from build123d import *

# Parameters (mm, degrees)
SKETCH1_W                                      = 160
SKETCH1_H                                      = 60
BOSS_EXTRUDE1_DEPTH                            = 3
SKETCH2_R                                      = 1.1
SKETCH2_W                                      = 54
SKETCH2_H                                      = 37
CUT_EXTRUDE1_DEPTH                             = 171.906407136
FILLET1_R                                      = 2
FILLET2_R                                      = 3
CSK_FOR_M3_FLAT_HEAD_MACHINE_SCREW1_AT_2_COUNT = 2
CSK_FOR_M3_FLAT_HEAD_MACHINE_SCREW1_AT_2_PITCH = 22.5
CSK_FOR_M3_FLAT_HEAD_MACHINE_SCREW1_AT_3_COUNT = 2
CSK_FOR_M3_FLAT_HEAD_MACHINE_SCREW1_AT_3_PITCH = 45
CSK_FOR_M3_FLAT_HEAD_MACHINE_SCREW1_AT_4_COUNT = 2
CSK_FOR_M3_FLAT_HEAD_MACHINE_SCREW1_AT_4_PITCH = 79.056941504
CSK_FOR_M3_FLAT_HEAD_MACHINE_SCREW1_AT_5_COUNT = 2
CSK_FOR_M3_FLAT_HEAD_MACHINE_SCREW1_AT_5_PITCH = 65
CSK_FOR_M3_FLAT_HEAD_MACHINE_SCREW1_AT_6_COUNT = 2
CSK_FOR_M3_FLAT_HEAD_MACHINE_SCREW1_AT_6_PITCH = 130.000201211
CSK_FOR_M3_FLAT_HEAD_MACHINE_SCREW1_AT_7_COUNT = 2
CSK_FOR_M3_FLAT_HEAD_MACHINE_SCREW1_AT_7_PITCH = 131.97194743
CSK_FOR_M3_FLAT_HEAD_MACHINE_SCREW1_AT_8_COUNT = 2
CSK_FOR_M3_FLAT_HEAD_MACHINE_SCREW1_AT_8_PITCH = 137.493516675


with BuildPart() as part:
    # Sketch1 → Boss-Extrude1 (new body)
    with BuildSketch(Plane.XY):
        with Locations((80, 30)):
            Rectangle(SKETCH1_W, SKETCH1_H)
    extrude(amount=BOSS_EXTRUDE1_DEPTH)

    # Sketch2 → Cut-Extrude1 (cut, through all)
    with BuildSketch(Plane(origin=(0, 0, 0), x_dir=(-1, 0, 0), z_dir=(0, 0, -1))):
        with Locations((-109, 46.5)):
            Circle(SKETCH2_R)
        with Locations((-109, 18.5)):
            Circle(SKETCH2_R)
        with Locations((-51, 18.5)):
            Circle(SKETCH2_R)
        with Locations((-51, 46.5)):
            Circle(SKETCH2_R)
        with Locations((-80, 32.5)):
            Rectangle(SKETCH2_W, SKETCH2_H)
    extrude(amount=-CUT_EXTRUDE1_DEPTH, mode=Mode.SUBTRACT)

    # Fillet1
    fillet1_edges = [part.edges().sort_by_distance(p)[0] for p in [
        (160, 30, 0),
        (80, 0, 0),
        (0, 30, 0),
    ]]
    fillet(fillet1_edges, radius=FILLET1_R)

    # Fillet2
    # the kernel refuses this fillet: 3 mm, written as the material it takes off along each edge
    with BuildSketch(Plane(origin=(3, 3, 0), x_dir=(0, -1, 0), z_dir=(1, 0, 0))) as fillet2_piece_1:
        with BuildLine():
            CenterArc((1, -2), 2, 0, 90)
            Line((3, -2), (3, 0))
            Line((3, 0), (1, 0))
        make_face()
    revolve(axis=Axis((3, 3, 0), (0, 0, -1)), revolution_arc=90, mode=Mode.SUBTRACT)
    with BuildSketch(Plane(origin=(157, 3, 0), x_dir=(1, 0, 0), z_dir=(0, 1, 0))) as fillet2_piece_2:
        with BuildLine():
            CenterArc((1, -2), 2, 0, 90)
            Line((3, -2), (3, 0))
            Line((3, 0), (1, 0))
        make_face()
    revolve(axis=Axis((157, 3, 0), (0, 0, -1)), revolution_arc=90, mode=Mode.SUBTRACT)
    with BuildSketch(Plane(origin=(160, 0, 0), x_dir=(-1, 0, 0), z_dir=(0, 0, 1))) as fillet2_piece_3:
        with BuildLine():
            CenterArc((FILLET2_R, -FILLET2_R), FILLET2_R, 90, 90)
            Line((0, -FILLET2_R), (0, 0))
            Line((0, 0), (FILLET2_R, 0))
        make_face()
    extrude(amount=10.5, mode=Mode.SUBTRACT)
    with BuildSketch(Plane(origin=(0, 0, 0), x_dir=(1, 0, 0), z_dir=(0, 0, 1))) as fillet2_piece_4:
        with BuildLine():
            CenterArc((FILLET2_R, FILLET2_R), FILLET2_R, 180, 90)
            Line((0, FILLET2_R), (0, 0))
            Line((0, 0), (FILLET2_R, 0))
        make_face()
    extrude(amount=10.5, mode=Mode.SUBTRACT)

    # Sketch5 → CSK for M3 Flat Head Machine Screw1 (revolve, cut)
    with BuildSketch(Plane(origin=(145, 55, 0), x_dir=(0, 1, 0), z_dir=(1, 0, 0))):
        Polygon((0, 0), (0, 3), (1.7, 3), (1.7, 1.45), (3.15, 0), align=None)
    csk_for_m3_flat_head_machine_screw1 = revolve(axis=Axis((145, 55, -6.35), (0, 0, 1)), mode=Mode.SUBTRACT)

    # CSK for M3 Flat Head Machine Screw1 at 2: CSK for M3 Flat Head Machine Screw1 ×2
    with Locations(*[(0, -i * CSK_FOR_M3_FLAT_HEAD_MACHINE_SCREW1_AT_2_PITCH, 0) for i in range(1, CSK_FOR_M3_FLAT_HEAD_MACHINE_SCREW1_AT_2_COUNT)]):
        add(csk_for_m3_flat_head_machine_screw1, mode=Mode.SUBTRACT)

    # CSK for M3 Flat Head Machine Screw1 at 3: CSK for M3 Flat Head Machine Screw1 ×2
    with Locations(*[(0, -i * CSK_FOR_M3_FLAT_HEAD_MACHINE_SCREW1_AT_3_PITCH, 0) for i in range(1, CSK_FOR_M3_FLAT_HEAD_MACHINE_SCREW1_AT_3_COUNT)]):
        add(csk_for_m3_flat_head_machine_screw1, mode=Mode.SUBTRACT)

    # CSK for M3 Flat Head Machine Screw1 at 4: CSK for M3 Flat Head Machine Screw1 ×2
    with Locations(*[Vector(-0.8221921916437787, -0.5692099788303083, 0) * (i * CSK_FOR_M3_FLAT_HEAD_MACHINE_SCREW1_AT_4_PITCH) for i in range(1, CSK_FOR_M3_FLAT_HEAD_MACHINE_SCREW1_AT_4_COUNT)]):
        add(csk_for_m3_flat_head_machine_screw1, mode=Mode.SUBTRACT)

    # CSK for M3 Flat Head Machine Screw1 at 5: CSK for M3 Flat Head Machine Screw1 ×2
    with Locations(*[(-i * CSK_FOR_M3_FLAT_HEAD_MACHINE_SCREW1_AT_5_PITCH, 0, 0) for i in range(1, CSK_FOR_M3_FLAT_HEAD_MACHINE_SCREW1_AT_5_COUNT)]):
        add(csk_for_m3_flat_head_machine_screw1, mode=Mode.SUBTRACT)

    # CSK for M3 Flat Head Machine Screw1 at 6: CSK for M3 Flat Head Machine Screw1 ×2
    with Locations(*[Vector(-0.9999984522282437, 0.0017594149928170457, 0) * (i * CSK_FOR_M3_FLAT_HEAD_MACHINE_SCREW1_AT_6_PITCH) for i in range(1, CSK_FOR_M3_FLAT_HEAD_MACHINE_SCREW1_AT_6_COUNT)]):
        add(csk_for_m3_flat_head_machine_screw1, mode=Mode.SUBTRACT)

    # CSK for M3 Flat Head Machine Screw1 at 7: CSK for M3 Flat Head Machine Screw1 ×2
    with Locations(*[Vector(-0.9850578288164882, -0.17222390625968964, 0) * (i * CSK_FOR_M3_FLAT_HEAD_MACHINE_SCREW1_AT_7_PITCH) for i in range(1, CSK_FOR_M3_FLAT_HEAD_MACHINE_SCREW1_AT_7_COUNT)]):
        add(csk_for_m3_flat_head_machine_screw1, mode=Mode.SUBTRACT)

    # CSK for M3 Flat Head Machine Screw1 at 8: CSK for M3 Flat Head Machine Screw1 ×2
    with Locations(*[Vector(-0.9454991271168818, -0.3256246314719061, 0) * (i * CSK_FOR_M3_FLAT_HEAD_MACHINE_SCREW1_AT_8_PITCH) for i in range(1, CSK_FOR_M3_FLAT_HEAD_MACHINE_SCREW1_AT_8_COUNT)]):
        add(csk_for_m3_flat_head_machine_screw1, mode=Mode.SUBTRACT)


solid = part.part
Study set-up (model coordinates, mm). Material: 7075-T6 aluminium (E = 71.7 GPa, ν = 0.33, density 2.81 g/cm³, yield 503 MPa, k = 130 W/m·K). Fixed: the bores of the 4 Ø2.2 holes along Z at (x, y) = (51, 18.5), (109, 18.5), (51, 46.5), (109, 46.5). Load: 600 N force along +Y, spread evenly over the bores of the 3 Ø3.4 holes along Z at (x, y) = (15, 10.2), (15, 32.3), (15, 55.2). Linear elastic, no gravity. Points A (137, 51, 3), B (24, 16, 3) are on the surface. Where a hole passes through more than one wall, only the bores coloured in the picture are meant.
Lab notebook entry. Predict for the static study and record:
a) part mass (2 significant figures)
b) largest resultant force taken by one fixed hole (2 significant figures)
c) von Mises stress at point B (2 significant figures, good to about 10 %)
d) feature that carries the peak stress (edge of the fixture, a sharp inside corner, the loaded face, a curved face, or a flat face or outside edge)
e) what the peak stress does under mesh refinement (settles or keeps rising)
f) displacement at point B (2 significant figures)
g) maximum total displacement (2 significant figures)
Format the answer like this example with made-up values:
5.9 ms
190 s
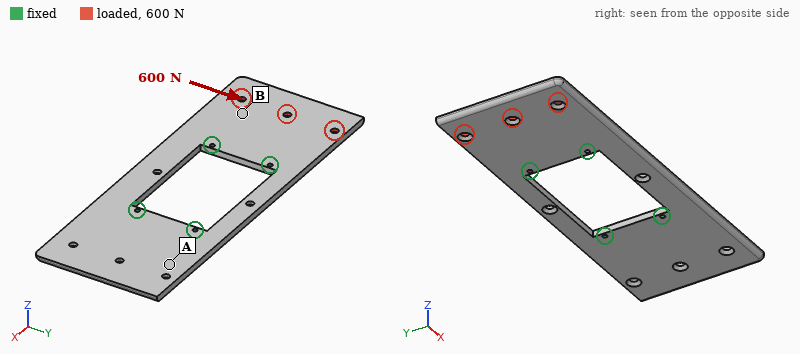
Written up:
62 g
600 N
9.4 MPa
edge of the fixture
keeps rising
15 µm
35 µm
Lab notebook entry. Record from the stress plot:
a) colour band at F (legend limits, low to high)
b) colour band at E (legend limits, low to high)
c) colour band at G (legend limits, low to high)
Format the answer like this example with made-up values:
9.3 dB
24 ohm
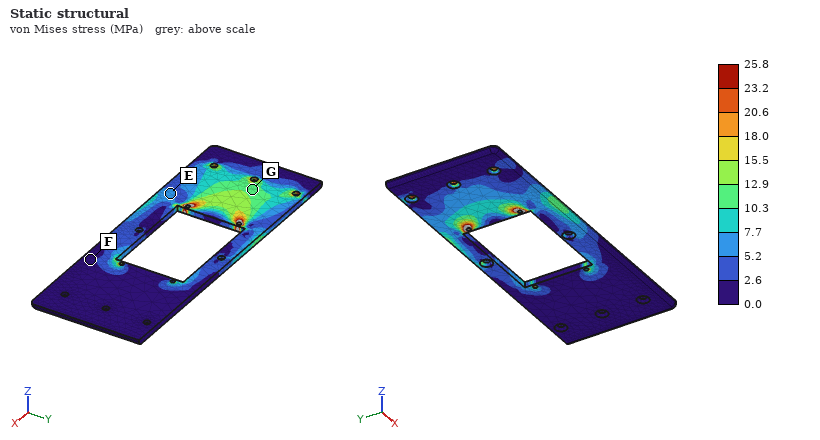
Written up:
0.0 to 2.6 MPa
5.2 to 7.7 MPa
10.3 to 12.9 MPa
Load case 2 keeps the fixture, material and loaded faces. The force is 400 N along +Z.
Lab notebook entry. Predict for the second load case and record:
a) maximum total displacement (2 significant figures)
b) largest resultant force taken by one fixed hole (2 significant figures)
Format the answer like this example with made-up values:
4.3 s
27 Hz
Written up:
1.4 mm
230 N
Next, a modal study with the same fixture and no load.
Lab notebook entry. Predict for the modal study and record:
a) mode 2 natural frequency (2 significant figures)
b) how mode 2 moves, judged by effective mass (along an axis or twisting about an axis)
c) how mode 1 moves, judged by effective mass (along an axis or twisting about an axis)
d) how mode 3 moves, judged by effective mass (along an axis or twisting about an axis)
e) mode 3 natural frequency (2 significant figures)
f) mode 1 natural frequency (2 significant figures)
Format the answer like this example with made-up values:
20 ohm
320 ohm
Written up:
840 Hz
twisting about Y
along Z
twisting about X
1800 Hz
810 Hz
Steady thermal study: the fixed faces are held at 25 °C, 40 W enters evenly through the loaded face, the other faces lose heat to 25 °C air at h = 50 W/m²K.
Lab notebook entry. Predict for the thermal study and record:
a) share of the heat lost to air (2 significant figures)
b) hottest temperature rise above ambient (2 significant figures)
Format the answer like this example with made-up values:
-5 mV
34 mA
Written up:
35 %
69 K
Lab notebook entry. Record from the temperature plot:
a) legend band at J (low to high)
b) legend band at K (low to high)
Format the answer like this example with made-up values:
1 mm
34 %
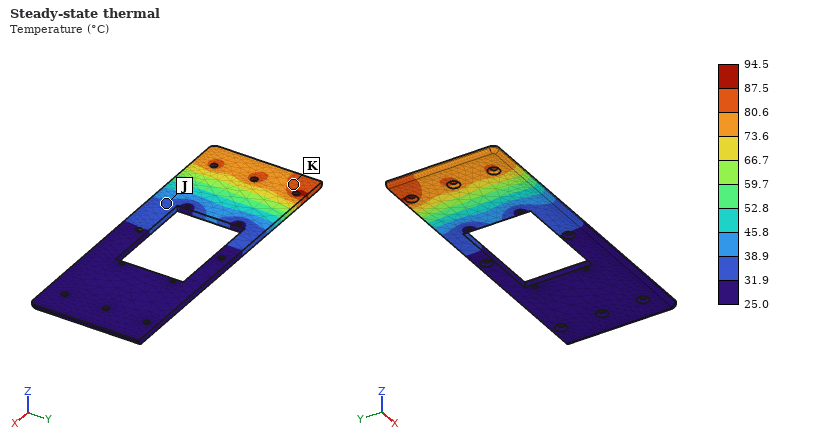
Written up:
31.9 to 38.9 °C
80.6 to 87.5 °C
